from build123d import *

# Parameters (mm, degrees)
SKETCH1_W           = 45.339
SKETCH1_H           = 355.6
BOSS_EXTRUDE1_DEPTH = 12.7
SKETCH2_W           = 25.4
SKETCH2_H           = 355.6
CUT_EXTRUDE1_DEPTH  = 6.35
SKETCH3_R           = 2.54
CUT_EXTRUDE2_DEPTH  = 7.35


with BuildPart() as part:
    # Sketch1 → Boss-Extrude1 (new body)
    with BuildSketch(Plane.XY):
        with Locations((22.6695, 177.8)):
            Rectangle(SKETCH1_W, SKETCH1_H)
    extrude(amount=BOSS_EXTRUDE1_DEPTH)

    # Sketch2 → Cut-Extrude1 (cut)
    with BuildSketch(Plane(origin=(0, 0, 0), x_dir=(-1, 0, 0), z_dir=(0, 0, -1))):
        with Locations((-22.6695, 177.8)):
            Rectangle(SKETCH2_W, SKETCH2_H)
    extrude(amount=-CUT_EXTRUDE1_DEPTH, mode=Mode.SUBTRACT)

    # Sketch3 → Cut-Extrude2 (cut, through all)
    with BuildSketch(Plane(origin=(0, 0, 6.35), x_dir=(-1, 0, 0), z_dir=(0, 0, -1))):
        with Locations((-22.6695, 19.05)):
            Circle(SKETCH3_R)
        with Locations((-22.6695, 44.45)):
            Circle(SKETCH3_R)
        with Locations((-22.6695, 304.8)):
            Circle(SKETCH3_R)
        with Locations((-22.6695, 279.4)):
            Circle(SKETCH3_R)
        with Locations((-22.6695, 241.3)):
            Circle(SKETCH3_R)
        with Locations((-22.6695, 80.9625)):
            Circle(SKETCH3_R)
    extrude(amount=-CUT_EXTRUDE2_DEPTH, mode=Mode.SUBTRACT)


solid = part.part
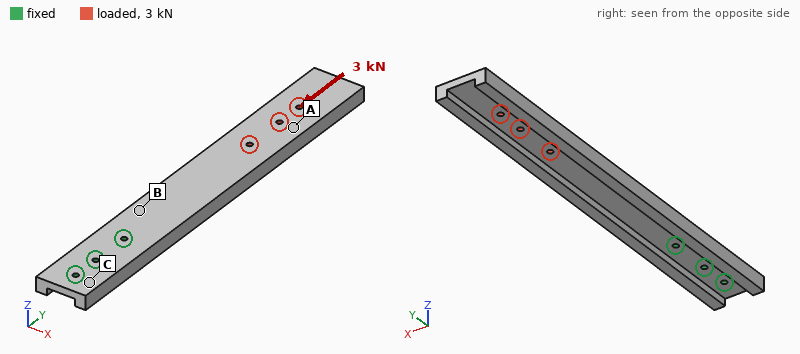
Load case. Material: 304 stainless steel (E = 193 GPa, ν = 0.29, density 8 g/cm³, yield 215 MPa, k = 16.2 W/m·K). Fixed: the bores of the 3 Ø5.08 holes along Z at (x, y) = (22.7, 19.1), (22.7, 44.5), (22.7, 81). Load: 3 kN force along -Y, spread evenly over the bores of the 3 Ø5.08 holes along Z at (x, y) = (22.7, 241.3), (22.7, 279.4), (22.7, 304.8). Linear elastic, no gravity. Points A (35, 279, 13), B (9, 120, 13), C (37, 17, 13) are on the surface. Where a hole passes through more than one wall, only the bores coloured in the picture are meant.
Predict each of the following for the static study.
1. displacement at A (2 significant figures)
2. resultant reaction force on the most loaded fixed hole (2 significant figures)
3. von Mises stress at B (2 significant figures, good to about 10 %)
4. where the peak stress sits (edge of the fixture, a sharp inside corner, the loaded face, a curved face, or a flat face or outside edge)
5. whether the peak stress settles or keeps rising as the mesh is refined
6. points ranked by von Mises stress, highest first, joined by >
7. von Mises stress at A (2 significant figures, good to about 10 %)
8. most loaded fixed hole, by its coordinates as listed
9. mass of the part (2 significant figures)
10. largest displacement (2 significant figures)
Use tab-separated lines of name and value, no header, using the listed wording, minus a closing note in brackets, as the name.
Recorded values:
displacement at A	0.12 mm
resultant reaction force on the most loaded fixed hole	2.1 kN
von Mises stress at B	13 MPa
where the peak stress sits	edge of the fixture
whether the peak stress settles or keeps rising as the mesh is refined	keeps rising
points ranked by von Mises stress, highest first, joined by >	B > A > C
von Mises stress at A	6.8 MPa
most loaded fixed hole, by its coordinates as listed	(22.7, 81)
mass of the part	1.2 kg
largest displacement	0.21 mm
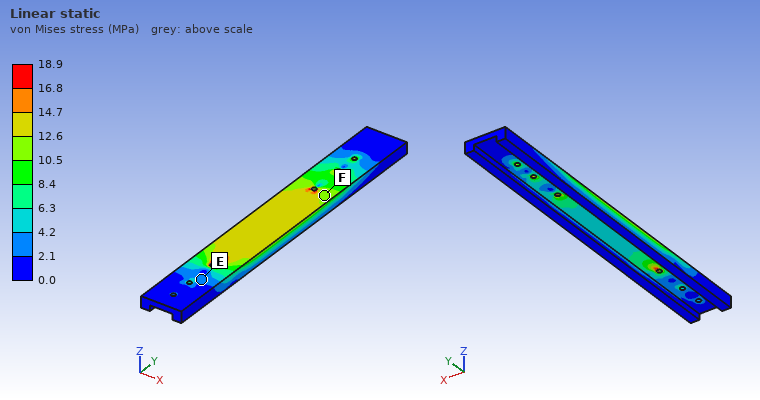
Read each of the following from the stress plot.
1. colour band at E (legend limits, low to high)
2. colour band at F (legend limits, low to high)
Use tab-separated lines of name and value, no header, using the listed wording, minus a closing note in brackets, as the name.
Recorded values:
colour band at E	2.1 to 4.2 MPa
colour band at F	10.5 to 12.6 MPa
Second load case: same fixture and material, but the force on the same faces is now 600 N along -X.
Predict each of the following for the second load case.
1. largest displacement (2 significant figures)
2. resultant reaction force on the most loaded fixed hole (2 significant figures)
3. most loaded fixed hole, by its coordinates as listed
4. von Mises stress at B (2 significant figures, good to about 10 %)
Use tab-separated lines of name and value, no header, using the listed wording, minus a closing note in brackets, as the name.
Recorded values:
largest displacement	0.21 mm
resultant reaction force on the most loaded fixed hole	2.8 kN
most loaded fixed hole, by its coordinates as listed	(22.7, 81)
von Mises stress at B	15 MPa
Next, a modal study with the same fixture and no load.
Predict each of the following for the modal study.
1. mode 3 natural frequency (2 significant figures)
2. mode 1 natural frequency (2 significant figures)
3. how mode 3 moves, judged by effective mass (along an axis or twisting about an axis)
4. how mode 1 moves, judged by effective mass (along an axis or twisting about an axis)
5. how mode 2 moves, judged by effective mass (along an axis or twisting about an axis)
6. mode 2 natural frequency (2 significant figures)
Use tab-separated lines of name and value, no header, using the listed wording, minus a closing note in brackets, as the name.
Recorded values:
mode 3 natural frequency	720 Hz
mode 1 natural frequency	120 Hz
how mode 3 moves, judged by effective mass	along Z
how mode 1 moves, judged by effective mass	along Z
how mode 2 moves, judged by effective mass	along X
mode 2 natural frequency	430 Hz
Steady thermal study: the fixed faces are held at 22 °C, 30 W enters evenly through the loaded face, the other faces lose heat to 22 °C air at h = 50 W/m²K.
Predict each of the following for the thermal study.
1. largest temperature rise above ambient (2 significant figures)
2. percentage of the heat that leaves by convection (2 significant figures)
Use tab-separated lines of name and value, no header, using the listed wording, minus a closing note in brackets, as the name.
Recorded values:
largest temperature rise above ambient	67 K
percentage of the heat that leaves by convection	100 %
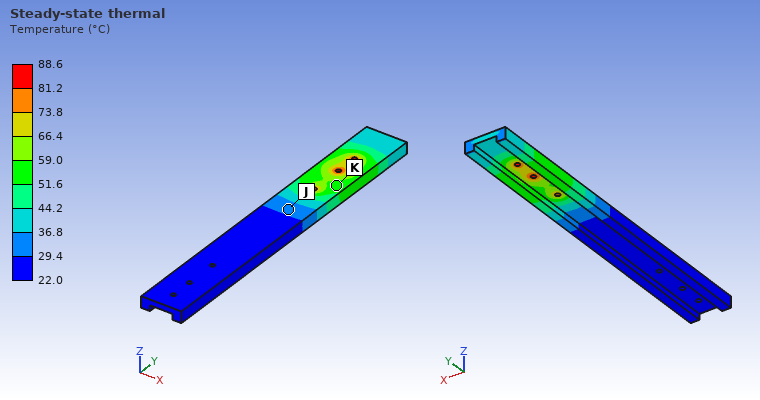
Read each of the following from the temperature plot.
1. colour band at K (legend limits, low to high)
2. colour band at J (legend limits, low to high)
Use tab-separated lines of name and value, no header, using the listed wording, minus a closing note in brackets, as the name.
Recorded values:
colour band at K	51.6 to 59.0 °C
colour band at J	29.4 to 36.8 °C
